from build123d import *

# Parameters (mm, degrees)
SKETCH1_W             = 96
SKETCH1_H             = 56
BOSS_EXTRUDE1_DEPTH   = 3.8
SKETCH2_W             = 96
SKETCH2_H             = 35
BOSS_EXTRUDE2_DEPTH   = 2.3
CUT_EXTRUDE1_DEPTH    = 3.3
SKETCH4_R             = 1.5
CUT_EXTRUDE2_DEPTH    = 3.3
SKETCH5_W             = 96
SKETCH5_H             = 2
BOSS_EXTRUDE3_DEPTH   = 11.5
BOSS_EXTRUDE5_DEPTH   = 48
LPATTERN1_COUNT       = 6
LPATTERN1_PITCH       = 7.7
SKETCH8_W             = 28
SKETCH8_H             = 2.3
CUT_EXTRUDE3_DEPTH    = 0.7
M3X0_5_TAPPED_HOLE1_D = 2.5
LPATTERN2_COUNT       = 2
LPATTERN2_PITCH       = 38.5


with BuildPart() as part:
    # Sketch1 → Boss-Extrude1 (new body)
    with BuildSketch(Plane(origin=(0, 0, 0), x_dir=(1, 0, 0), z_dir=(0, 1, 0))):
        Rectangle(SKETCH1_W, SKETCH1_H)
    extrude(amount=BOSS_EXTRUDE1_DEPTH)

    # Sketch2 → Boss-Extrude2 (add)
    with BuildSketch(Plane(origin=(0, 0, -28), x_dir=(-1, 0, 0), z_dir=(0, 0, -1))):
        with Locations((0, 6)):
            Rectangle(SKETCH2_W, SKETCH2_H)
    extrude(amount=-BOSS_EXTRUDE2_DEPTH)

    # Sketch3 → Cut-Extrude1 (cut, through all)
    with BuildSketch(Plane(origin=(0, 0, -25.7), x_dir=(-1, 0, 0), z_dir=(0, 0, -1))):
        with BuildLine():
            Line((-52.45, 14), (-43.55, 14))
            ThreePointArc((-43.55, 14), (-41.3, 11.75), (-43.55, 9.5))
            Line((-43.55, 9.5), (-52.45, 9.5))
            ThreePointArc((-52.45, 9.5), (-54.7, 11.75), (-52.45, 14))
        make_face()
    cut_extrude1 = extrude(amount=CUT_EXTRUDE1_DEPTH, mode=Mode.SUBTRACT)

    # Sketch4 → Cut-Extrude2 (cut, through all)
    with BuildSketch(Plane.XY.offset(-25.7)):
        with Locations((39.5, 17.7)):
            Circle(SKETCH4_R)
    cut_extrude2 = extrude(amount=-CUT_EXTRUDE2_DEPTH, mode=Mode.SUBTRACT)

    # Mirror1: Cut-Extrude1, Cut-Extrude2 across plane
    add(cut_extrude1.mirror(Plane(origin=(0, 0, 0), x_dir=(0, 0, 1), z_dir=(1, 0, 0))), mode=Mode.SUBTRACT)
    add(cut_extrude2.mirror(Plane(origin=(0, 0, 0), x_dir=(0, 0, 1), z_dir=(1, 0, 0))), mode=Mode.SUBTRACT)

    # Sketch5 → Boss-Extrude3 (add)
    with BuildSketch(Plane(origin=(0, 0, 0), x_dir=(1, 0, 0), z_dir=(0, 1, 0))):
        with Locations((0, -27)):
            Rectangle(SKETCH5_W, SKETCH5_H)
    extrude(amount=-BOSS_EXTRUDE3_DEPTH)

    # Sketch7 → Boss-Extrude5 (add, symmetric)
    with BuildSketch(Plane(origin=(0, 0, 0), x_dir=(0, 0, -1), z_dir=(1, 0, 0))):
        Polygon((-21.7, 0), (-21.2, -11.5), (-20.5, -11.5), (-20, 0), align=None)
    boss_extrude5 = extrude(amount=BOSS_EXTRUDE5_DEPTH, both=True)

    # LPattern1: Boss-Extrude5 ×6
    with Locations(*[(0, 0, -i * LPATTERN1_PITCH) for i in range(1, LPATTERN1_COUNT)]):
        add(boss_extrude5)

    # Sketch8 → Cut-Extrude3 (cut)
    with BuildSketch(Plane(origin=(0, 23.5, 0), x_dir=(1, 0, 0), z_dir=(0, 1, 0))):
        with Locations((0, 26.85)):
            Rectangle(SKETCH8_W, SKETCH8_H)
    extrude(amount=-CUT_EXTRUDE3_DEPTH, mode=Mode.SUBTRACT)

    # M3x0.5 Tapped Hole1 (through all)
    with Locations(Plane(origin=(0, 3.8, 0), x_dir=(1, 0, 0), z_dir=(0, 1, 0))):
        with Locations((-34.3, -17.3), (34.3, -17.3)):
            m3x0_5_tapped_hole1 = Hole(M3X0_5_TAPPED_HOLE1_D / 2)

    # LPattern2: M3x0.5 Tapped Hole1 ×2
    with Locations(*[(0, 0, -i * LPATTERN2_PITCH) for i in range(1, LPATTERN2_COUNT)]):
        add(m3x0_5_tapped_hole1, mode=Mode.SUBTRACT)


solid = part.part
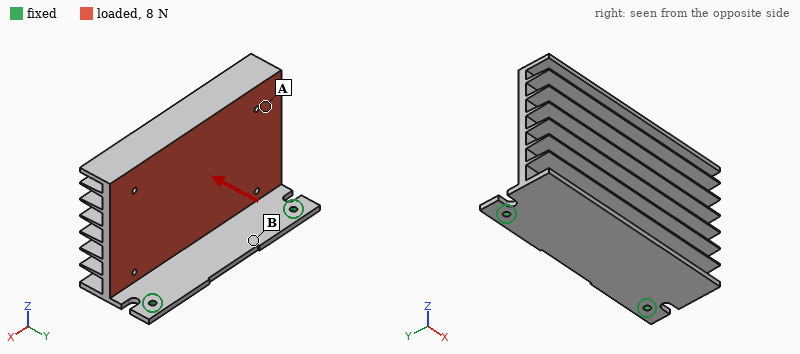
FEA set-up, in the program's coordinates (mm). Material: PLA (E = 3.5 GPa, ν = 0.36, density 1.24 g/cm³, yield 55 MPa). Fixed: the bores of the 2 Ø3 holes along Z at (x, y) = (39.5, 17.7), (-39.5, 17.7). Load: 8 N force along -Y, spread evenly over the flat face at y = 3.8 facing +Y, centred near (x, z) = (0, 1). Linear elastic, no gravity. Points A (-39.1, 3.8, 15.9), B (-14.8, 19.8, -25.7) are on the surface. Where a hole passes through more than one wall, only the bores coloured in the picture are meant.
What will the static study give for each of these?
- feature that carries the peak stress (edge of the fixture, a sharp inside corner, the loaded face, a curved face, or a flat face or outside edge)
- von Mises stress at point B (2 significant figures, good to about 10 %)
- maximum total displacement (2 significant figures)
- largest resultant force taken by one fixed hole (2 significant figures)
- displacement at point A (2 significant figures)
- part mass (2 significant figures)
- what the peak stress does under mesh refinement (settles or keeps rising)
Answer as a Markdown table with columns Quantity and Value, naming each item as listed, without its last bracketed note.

| Quantity | Value |
|---|---|
| feature that carries the peak stress | edge of the fixture |
| von Mises stress at point B | 1.9 MPa |
| maximum total displacement | 1.3 mm |
| largest resultant force taken by one fixed hole | 4.5 N |
| displacement at point A | 0.98 mm |
| part mass | 46 g |
| what the peak stress does under mesh refinement | keeps rising |
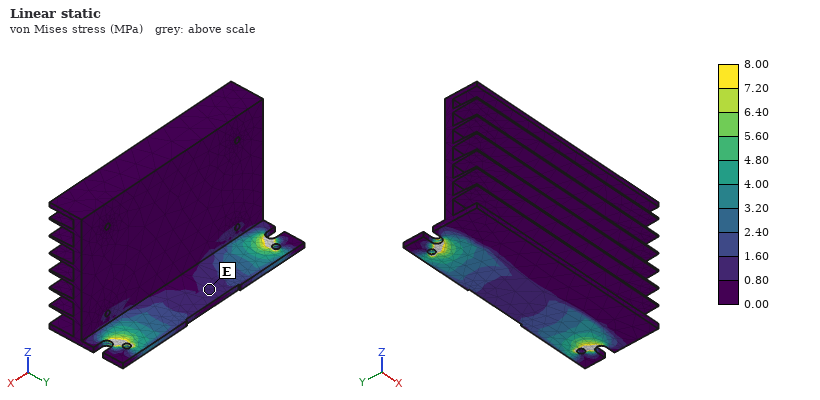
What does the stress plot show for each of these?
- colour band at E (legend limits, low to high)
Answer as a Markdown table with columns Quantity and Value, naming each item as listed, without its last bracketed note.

| Quantity | Value |
|---|---|
| colour band at E | 0.80 to 1.60 MPa |
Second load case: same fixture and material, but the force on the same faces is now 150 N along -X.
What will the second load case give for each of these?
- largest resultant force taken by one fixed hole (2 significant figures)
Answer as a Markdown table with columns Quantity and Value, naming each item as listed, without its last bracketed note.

| Quantity | Value |
|---|---|
| largest resultant force taken by one fixed hole | 97 N |
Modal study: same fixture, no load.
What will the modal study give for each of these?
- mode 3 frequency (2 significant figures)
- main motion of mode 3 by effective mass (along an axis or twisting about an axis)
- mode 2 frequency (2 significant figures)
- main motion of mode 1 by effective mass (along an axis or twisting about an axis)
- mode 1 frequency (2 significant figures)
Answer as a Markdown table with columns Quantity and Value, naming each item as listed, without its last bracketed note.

| Quantity | Value |
|---|---|
| mode 3 frequency | 440 Hz |
| main motion of mode 3 by effective mass | along X |
| mode 2 frequency | 290 Hz |
| main motion of mode 1 by effective mass | along Y |
| mode 1 frequency | 72 Hz |
